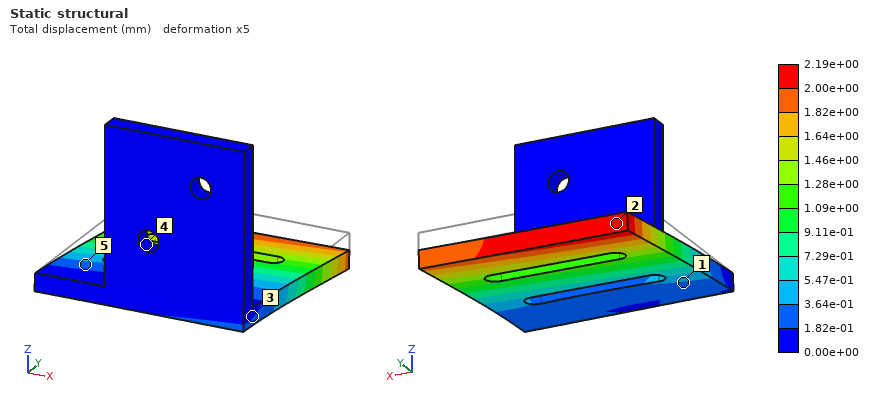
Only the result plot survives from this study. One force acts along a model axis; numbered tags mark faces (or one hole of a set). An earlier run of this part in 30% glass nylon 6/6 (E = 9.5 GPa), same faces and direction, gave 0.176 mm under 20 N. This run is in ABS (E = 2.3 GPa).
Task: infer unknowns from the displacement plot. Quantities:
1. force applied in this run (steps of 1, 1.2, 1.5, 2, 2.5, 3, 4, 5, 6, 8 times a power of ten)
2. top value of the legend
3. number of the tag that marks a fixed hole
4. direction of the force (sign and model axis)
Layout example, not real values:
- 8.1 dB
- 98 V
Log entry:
- 60 N
- 2.19e+00 mm
- 4
- -Z
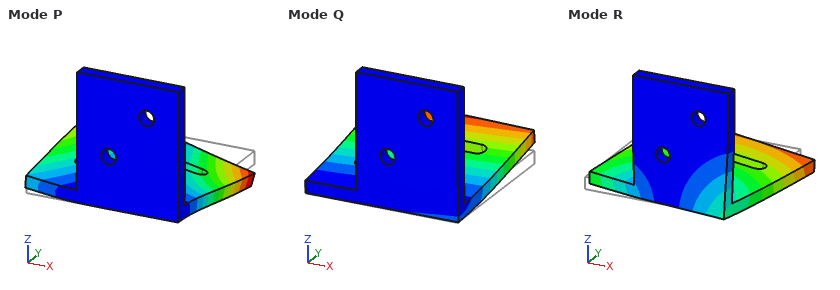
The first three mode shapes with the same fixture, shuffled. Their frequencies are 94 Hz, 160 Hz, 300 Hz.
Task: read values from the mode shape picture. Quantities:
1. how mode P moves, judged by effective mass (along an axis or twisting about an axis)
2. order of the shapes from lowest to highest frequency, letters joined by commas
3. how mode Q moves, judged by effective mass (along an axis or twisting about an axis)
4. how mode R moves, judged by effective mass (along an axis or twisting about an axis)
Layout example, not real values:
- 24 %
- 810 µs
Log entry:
- twisting about Y
- Q, R, P
- along Z
- along X
